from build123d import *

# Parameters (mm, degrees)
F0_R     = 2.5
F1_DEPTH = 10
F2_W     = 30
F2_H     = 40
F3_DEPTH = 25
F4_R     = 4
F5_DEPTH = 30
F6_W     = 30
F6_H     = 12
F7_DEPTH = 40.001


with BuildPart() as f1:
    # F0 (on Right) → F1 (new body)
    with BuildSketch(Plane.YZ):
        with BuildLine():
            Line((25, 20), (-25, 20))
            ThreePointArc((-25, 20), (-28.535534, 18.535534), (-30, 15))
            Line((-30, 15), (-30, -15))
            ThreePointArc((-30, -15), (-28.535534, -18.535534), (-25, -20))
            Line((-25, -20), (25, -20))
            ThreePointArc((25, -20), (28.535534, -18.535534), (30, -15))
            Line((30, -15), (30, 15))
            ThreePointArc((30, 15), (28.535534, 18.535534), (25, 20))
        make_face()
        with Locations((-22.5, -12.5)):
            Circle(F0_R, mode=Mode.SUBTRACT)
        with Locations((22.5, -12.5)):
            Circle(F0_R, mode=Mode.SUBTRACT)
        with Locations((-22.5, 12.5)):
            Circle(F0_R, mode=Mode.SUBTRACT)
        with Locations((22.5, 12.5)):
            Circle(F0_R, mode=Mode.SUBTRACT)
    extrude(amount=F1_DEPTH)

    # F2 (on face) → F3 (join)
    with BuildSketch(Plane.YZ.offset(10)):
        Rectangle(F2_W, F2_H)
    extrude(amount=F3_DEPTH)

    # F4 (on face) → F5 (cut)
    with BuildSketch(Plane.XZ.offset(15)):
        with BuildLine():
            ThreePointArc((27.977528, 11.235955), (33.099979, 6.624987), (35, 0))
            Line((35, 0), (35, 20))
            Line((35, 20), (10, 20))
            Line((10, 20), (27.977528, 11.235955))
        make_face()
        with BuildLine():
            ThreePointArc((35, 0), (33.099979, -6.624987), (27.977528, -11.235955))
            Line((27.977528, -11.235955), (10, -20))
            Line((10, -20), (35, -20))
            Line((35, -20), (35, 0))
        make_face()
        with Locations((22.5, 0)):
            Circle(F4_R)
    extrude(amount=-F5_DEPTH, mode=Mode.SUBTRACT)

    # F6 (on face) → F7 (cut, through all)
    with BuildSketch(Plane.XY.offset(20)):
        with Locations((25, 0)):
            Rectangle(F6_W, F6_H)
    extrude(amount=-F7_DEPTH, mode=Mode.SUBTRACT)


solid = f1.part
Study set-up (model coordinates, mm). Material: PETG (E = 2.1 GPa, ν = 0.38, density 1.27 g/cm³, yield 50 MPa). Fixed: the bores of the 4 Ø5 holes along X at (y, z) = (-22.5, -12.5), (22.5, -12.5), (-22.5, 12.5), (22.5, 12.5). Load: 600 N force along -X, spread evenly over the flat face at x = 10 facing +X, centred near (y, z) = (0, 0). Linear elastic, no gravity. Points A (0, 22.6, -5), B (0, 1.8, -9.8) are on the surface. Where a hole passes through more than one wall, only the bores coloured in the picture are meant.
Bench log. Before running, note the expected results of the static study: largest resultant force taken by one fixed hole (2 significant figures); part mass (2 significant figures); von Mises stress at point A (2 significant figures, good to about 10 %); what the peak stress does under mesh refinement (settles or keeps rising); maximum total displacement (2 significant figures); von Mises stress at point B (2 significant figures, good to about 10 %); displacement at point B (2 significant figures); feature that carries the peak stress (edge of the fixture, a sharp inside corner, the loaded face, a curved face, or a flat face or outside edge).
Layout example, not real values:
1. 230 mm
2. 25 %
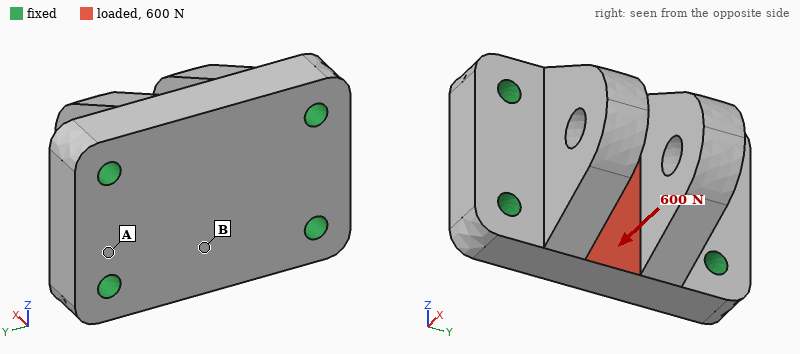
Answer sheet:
1. 150 N
2. 43 g
3. 1.3 MPa
4. keeps rising
5. 0.10 mm
6. 3.4 MPa
7. 0.055 mm
8. edge of the fixture
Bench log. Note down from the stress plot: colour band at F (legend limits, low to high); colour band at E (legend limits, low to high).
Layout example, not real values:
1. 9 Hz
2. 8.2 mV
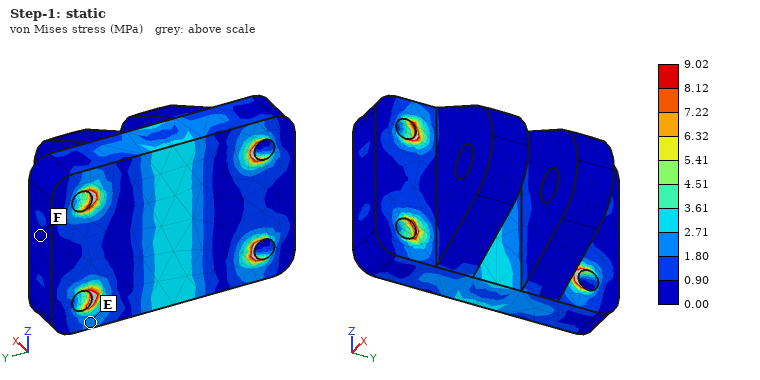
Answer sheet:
1. 0.00 to 0.90 MPa
2. 1.80 to 2.71 MPa
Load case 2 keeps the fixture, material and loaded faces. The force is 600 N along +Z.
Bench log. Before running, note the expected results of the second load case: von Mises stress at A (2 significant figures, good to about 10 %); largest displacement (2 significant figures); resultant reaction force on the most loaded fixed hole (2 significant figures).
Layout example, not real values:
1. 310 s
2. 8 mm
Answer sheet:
1. 0.45 MPa
2. 42 µm
3. 190 N
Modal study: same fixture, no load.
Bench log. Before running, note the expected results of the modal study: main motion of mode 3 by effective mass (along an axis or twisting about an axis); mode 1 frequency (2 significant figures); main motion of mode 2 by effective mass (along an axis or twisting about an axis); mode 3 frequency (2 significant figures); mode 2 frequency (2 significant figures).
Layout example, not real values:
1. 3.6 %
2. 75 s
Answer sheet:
1. along Z
2. 2500 Hz
3. along Y
4. 3600 Hz
5. 3000 Hz
